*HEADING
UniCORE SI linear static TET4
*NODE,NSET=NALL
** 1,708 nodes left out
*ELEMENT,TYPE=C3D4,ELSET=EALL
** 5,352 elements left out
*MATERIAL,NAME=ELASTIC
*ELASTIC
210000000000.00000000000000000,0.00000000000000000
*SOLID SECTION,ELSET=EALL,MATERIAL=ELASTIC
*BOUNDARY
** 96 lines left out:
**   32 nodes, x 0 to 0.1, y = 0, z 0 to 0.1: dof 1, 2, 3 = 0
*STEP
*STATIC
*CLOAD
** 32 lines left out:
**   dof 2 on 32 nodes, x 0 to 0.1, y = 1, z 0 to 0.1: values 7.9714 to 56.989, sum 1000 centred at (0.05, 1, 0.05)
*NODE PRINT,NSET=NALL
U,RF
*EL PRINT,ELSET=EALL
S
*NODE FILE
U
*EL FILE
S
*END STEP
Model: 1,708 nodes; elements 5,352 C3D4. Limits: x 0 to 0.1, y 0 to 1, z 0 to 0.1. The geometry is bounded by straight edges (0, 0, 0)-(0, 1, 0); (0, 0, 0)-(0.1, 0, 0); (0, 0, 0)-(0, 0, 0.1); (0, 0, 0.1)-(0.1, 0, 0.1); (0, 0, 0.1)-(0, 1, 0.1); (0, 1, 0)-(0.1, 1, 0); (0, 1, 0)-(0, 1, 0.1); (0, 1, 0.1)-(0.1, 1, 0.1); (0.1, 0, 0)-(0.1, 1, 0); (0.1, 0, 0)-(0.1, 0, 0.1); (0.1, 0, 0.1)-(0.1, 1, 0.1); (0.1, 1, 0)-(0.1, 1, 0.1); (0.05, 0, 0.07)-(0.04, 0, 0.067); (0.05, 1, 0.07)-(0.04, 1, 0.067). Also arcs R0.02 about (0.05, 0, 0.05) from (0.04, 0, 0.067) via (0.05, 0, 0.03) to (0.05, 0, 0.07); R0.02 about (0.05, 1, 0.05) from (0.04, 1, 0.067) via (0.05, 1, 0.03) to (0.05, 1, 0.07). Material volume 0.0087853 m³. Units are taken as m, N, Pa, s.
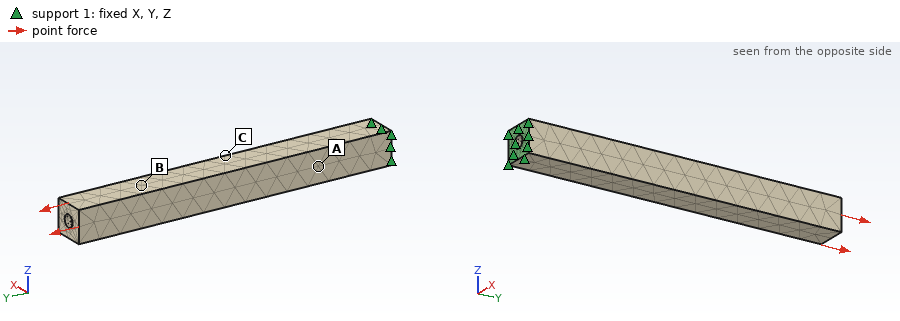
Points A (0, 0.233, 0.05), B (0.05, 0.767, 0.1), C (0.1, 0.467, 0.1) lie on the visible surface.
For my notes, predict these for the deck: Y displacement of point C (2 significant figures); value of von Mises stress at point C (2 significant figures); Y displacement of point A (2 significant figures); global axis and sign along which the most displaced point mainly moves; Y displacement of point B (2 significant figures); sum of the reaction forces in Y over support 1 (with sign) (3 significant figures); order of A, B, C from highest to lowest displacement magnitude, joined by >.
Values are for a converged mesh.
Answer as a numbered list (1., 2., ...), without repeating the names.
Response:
1. 2.5e-07 m
2. 1.1e+05 Pa
3. 1.3e-07 m
4. +Y
5. 4.2e-07 m
6. -1000 N
7. B > C > A
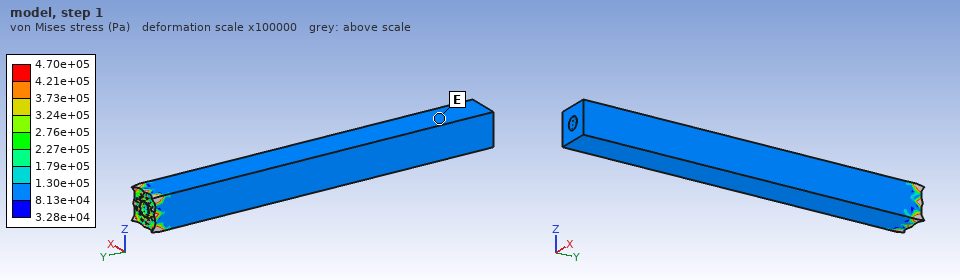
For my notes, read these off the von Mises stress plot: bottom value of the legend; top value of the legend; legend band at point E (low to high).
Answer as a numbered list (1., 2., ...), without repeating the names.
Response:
1. 3.28e+04 Pa
2. 4.70e+05 Pa
3. 8.13e+04 to 1.30e+05 Pa
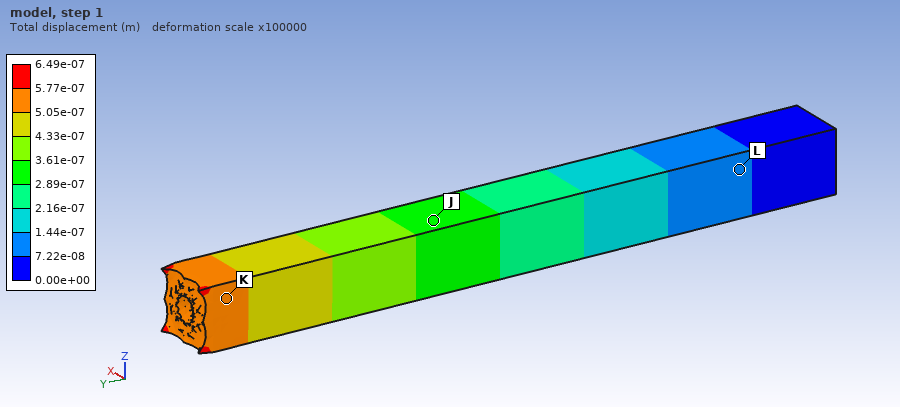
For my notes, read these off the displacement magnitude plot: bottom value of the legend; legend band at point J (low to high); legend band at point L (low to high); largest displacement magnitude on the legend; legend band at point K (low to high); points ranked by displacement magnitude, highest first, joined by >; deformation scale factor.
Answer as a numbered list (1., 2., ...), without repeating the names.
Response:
1. 0.00e+00 m
2. 2.89e-07 to 3.61e-07 m
3. 7.22e-08 to 1.44e-07 m
4. 6.49e-07 m
5. 5.05e-07 to 5.77e-07 m
6. K > J > L
7. 100000
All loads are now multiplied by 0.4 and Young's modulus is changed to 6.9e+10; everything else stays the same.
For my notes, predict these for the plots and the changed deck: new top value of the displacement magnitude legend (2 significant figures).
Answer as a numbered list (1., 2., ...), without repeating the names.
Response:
1. 7.9e-07 m
